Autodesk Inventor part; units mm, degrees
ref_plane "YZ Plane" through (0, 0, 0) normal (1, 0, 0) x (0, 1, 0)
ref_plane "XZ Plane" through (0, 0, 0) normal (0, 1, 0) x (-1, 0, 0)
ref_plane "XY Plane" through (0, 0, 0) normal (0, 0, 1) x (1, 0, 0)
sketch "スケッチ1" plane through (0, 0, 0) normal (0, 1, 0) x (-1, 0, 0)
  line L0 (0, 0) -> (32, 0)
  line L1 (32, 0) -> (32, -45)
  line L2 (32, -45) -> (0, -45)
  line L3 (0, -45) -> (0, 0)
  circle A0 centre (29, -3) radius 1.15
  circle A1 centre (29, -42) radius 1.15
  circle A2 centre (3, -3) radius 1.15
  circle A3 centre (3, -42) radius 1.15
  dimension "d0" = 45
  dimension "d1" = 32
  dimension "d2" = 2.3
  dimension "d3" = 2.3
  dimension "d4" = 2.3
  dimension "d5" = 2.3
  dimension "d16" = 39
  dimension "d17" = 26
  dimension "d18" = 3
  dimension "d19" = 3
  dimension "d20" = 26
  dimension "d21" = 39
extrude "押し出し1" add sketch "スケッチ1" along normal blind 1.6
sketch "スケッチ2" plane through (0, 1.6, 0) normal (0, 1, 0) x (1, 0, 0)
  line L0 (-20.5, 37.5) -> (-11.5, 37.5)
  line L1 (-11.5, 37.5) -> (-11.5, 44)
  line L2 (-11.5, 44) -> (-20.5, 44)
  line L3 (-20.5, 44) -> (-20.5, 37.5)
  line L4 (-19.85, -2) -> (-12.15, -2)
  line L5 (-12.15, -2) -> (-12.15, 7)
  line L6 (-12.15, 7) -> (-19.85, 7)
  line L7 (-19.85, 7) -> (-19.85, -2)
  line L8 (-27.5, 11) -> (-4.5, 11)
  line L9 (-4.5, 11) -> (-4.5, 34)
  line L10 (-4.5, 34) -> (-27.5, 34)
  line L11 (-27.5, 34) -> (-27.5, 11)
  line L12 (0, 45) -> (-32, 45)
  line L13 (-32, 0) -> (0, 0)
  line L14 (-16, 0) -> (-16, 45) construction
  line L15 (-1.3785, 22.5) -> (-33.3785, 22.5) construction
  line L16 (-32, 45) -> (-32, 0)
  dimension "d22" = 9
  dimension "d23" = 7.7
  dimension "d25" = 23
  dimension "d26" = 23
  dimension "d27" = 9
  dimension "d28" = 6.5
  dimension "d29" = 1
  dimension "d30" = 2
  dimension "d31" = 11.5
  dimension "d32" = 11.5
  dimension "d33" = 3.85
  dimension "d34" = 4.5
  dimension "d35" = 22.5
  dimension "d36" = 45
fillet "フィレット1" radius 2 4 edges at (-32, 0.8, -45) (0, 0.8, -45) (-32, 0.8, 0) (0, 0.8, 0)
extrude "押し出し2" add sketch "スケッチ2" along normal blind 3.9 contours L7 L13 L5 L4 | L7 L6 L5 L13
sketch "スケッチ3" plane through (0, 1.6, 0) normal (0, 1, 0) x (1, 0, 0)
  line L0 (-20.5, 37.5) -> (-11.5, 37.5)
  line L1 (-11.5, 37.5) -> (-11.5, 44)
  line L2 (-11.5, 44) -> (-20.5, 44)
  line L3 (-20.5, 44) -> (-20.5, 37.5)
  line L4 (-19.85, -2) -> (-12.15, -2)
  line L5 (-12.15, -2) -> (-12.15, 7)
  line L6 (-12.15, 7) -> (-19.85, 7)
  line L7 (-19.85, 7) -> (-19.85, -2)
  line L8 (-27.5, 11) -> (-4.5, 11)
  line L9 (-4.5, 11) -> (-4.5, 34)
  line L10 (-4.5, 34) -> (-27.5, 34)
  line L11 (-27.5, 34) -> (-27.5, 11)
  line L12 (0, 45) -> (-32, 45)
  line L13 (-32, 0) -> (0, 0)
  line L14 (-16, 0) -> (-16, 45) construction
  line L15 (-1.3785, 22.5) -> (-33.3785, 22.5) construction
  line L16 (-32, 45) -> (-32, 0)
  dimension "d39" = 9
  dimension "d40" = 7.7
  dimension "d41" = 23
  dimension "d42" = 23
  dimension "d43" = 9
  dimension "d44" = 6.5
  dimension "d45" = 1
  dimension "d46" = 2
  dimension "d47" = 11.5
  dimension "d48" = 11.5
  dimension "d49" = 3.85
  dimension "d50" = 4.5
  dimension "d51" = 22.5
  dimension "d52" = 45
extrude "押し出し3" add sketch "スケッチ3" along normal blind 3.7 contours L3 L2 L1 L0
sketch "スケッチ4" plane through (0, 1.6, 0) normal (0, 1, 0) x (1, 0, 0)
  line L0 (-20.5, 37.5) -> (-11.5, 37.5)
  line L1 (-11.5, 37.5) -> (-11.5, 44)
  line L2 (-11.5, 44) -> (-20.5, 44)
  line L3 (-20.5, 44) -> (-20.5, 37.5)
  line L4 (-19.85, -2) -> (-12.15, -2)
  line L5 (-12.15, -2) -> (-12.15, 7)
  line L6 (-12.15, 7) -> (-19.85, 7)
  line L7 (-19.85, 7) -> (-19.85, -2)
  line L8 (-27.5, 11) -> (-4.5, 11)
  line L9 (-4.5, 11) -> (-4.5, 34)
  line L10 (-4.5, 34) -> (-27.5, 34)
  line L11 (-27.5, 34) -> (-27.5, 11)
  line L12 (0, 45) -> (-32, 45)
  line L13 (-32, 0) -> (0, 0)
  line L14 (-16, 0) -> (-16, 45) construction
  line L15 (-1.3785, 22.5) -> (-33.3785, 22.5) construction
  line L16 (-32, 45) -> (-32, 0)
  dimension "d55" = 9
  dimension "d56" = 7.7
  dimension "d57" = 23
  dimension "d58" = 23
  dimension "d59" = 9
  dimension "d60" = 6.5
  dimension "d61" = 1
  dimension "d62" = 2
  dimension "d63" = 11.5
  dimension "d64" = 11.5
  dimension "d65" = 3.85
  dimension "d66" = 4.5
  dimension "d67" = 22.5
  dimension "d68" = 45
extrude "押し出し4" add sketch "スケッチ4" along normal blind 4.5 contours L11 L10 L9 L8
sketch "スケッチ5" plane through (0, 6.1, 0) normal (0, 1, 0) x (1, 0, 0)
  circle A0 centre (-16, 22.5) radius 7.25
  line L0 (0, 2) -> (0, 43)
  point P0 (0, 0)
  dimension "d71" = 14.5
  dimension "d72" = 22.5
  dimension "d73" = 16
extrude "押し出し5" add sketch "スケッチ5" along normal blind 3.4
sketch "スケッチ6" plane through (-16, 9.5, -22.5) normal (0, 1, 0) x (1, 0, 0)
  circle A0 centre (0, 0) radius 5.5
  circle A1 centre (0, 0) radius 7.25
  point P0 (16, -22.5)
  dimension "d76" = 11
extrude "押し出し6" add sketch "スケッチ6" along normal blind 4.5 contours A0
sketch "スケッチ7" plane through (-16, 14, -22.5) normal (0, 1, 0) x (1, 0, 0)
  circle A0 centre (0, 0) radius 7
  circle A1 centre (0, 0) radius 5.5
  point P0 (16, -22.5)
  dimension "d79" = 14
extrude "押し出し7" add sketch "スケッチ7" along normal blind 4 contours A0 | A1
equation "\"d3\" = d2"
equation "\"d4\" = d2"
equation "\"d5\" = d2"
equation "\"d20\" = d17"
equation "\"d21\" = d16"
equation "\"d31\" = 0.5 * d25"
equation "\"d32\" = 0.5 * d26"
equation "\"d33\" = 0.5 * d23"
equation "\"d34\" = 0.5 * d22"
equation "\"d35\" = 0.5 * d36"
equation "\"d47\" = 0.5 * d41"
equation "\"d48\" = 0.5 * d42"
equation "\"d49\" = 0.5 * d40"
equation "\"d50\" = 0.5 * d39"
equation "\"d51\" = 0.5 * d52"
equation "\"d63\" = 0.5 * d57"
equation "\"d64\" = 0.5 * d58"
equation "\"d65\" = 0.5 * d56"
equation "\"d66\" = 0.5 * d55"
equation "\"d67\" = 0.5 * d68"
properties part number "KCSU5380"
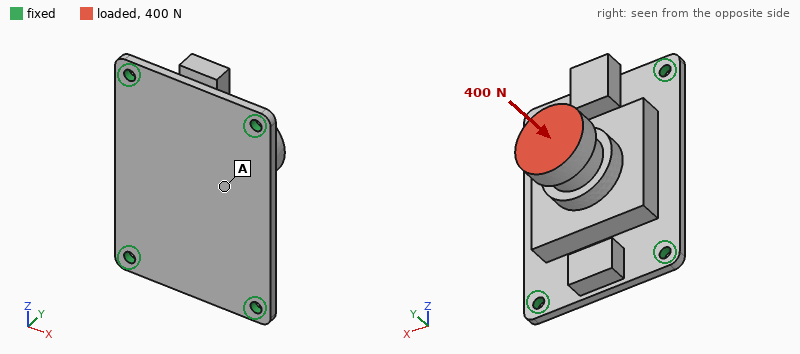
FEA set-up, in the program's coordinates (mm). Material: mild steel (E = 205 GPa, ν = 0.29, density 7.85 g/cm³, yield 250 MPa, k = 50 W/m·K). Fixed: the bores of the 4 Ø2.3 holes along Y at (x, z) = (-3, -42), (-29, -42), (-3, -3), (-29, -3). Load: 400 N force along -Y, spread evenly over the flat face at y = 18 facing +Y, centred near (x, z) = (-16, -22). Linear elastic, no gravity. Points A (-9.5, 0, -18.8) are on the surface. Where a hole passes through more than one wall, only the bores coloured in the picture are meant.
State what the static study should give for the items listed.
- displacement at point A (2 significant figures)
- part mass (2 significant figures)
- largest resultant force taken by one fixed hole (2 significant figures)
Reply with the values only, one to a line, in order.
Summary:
11 µm
53 g
130 N
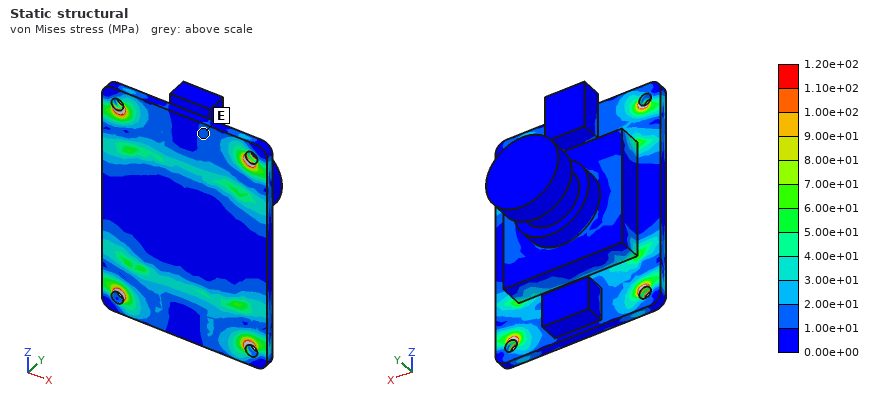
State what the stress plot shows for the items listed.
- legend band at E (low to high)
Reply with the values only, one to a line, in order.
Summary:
1.00e+01 to 2.00e+01 MPa
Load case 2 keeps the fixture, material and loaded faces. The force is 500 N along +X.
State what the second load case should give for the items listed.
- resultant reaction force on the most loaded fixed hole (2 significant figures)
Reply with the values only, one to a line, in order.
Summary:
270 N
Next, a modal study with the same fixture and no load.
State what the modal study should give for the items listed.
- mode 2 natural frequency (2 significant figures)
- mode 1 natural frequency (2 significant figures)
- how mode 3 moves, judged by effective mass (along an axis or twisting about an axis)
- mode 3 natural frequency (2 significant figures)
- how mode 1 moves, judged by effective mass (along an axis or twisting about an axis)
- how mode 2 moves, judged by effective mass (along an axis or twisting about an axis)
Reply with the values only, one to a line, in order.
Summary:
5900 Hz
4700 Hz
along Z
7700 Hz
along Y
along X
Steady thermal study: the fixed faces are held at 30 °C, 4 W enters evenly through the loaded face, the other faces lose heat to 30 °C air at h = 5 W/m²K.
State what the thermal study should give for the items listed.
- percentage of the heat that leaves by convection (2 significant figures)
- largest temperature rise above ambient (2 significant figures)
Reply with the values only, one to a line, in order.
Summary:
5.0 %
22 K
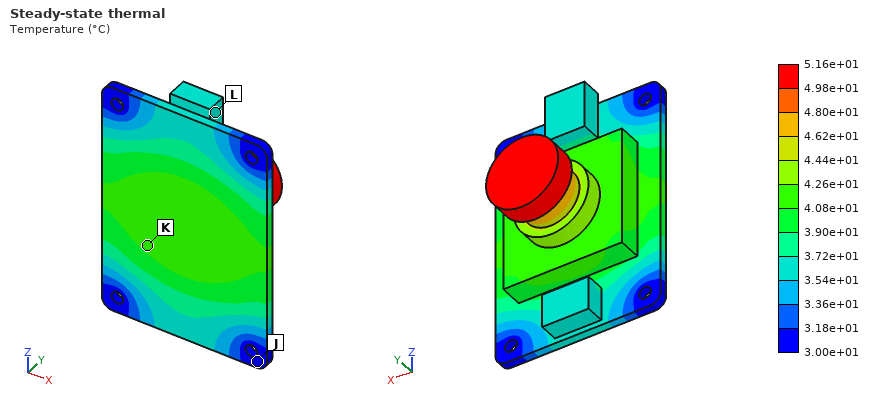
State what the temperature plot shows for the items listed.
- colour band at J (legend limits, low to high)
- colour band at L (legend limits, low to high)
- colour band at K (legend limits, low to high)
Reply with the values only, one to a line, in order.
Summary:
3.00e+01 to 3.18e+01 °C
3.54e+01 to 3.72e+01 °C
4.08e+01 to 4.26e+01 °C
